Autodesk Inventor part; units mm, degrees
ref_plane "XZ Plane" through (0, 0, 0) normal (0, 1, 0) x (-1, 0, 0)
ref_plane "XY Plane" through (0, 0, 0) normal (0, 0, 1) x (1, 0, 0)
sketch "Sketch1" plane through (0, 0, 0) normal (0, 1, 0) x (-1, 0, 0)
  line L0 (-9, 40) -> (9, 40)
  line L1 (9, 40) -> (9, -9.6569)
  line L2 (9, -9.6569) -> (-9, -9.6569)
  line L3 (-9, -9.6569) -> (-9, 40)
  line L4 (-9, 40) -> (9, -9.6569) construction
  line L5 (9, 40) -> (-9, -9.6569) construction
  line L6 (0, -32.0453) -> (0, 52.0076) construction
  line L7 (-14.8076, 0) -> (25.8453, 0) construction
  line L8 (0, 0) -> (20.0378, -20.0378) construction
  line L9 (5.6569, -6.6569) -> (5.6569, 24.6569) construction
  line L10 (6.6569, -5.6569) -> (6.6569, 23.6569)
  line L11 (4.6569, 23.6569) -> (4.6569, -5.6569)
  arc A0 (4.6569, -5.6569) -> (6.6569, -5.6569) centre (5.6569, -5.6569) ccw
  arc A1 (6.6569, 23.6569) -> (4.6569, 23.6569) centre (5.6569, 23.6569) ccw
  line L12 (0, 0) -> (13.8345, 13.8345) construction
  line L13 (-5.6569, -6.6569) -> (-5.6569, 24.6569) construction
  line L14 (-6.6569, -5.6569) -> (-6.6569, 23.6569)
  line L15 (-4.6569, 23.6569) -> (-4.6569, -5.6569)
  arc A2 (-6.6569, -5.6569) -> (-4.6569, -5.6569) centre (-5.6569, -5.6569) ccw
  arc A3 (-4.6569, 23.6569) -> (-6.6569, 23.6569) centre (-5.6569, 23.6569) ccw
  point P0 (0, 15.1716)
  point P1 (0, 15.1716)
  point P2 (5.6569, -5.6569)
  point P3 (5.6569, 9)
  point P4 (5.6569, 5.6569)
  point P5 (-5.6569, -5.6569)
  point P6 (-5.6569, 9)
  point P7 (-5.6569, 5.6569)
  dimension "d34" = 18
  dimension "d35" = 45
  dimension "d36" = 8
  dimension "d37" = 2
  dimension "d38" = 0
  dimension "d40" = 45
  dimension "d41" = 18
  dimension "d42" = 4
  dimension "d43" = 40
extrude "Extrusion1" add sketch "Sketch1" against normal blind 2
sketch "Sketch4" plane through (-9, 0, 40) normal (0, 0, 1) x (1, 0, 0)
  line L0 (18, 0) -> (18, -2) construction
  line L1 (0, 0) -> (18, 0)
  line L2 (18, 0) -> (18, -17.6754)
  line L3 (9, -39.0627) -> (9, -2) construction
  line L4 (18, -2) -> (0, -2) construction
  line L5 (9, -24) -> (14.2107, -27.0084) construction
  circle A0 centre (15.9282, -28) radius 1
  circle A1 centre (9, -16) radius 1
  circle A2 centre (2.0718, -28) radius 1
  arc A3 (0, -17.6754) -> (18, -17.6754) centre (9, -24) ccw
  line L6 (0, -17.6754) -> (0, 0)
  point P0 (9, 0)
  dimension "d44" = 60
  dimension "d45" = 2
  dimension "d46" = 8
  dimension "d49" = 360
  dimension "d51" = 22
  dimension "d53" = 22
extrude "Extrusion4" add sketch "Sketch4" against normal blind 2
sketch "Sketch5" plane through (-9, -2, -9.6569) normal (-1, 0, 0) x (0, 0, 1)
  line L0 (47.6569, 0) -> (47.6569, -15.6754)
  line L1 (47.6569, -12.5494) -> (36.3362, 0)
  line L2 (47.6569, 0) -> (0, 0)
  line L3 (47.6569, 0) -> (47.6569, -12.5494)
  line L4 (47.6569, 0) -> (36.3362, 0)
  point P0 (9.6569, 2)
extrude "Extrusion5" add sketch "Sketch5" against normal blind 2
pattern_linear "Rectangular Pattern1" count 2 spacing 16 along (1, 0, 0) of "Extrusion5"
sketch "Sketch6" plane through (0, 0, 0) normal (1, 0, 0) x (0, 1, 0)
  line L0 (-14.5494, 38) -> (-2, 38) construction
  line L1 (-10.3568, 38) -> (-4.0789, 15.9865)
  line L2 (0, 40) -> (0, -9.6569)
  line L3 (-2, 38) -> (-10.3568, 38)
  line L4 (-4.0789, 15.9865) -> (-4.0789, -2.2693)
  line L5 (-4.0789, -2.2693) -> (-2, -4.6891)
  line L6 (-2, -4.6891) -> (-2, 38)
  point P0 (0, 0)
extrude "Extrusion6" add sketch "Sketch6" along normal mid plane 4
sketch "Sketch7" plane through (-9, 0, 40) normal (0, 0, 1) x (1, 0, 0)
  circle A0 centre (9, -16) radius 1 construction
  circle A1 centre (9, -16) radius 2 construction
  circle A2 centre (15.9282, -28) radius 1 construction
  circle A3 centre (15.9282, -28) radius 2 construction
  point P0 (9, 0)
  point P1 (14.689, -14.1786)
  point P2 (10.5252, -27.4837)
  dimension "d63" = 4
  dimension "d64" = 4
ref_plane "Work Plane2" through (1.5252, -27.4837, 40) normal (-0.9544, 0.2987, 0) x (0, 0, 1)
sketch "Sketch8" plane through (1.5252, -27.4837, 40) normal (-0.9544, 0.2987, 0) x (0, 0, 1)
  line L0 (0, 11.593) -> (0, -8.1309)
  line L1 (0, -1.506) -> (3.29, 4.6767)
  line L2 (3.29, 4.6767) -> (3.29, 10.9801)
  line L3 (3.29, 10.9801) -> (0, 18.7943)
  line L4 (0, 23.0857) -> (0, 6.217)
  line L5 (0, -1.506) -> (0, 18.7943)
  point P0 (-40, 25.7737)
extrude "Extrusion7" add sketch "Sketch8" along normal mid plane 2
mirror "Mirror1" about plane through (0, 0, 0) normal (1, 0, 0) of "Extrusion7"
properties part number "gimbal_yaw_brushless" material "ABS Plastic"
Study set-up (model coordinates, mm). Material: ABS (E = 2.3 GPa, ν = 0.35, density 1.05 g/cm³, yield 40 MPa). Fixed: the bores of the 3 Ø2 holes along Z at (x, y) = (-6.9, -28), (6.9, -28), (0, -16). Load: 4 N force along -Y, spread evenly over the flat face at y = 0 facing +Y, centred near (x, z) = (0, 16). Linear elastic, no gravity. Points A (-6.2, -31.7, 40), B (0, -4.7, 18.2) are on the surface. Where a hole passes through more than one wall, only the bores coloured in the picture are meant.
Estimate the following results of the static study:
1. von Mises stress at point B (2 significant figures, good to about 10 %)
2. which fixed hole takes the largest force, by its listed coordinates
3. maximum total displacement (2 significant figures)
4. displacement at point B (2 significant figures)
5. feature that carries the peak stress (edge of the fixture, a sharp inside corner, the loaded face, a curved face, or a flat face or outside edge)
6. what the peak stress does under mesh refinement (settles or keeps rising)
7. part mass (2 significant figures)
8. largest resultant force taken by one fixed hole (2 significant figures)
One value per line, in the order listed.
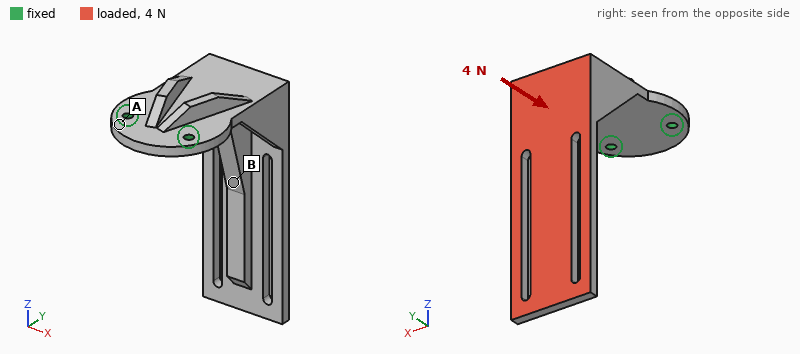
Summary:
1.6 MPa
(0, -16)
0.68 mm
0.25 mm
edge of the fixture
keeps rising
4.0 g
7.5 N
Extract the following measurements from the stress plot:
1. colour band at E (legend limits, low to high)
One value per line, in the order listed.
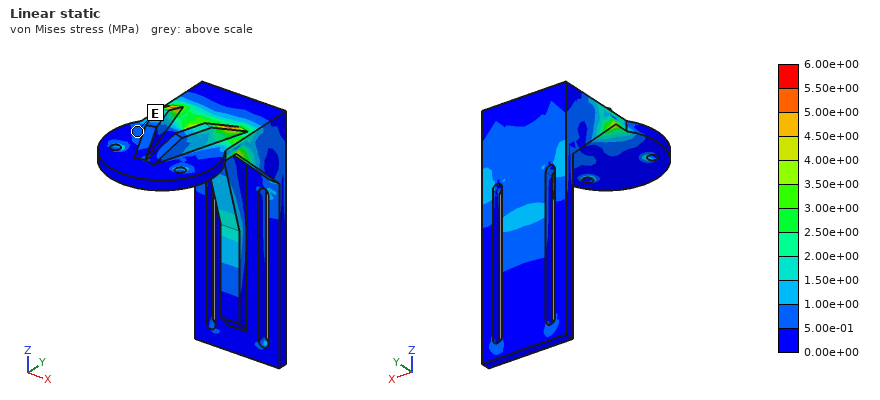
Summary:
5.00e-01 to 1.00e+00 MPa
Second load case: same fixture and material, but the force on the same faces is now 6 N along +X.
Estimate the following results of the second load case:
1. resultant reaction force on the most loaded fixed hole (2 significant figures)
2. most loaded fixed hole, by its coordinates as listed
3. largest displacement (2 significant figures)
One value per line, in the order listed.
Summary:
12 N
(0, -16)
0.70 mm
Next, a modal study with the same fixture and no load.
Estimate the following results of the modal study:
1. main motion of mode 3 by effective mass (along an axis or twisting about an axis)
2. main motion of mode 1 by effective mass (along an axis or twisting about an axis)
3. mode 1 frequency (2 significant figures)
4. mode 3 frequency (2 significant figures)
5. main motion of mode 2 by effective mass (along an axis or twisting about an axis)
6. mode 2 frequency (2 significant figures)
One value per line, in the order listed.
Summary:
along Z
along Y
320 Hz
1400 Hz
along X
400 Hz
